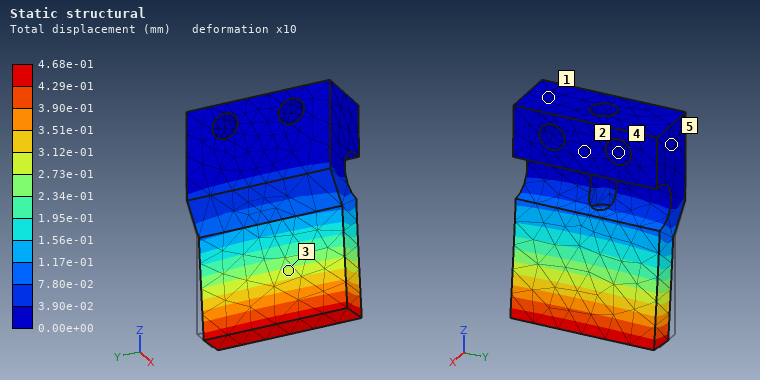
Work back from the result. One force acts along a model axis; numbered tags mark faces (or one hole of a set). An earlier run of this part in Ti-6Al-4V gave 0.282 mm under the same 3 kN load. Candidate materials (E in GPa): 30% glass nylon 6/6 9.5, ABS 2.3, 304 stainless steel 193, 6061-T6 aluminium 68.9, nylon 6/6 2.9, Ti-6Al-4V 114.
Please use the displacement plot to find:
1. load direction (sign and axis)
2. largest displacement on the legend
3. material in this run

+X
4.68e-01 mm
6061-T6 aluminium
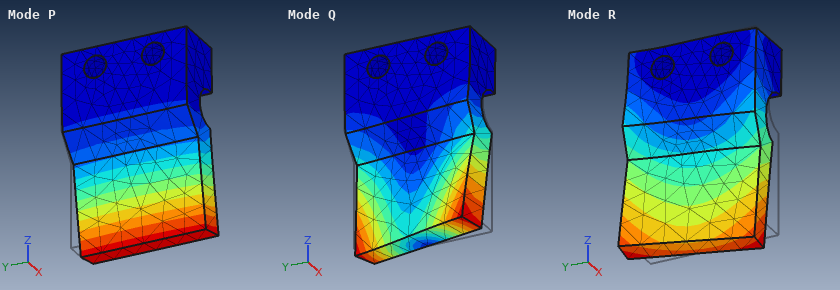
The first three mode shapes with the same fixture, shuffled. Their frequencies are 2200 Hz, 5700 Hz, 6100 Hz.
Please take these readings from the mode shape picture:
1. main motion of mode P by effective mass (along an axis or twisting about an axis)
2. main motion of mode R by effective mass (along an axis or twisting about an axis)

along X
along Y
